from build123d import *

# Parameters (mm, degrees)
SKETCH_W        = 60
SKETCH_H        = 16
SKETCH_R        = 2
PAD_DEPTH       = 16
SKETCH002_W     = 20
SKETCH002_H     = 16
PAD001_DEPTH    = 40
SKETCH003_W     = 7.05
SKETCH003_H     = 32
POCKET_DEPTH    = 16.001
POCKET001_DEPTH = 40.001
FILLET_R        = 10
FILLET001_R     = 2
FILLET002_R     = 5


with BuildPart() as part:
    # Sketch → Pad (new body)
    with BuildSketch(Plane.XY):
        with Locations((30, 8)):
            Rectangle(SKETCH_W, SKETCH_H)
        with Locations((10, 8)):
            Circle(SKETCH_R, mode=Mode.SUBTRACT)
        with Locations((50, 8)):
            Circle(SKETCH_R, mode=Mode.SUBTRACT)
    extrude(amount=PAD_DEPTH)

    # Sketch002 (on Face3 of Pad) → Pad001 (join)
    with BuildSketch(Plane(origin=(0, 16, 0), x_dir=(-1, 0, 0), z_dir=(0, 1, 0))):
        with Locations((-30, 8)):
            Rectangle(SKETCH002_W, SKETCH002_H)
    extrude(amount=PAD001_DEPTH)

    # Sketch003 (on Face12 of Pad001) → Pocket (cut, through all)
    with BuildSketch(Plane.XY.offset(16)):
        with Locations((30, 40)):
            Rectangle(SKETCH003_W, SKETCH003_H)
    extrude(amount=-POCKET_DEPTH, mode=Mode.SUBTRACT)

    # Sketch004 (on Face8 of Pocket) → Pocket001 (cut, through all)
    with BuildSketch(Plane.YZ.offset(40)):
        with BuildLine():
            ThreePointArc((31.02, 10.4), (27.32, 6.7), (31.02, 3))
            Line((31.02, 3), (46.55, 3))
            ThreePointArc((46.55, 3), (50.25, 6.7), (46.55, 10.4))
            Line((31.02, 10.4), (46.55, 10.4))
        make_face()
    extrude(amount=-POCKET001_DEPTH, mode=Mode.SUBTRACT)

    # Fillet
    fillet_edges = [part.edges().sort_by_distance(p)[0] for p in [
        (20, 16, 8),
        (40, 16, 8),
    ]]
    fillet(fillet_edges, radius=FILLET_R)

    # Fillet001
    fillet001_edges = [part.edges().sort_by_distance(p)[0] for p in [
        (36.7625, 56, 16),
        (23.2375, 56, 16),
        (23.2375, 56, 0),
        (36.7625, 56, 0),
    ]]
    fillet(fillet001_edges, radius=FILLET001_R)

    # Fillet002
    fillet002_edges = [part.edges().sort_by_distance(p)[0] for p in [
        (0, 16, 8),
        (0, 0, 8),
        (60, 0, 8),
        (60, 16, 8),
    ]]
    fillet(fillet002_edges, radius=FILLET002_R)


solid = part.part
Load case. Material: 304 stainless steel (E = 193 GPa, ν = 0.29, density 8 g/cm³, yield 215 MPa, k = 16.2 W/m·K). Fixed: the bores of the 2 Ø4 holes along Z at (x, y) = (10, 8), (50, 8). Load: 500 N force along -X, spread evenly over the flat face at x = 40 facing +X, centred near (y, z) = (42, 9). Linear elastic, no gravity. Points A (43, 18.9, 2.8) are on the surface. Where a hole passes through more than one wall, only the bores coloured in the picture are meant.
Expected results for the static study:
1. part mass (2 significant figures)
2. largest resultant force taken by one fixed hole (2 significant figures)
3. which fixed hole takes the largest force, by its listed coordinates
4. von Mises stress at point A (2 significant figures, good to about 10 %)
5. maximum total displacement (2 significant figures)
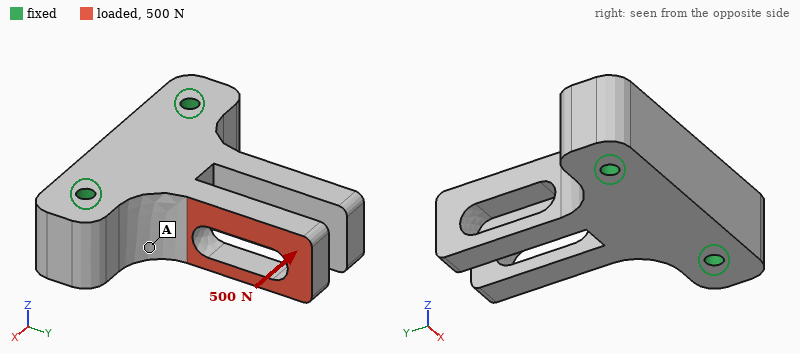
180 g
550 N
(10, 8)
16 MPa
72 µm
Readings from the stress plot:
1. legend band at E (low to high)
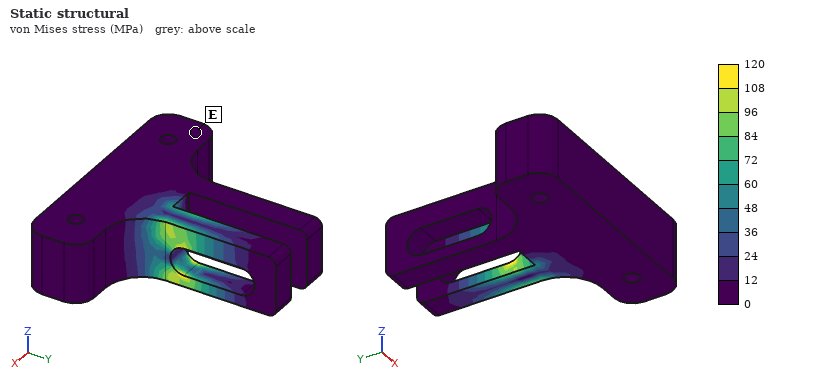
0 to 12 MPa
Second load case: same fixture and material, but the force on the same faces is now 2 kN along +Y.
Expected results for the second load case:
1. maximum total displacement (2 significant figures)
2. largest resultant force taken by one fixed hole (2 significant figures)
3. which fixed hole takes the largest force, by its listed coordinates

68 µm
1.6 kN
(50, 8)
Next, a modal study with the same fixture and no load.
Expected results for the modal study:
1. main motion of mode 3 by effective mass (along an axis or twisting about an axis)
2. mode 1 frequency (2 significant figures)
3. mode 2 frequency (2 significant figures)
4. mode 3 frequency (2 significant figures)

along Z
3900 Hz
3900 Hz
4600 Hz
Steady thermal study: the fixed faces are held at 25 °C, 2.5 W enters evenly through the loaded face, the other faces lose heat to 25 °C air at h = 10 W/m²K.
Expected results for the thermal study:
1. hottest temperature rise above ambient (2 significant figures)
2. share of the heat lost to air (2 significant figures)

48 K
21 %
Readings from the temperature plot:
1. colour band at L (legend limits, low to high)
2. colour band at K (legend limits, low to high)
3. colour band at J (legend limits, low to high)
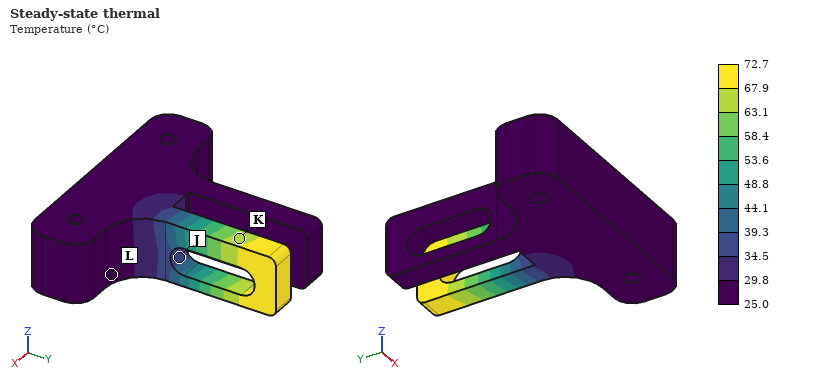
25.0 to 29.8 °C
63.1 to 67.9 °C
34.5 to 39.3 °C
